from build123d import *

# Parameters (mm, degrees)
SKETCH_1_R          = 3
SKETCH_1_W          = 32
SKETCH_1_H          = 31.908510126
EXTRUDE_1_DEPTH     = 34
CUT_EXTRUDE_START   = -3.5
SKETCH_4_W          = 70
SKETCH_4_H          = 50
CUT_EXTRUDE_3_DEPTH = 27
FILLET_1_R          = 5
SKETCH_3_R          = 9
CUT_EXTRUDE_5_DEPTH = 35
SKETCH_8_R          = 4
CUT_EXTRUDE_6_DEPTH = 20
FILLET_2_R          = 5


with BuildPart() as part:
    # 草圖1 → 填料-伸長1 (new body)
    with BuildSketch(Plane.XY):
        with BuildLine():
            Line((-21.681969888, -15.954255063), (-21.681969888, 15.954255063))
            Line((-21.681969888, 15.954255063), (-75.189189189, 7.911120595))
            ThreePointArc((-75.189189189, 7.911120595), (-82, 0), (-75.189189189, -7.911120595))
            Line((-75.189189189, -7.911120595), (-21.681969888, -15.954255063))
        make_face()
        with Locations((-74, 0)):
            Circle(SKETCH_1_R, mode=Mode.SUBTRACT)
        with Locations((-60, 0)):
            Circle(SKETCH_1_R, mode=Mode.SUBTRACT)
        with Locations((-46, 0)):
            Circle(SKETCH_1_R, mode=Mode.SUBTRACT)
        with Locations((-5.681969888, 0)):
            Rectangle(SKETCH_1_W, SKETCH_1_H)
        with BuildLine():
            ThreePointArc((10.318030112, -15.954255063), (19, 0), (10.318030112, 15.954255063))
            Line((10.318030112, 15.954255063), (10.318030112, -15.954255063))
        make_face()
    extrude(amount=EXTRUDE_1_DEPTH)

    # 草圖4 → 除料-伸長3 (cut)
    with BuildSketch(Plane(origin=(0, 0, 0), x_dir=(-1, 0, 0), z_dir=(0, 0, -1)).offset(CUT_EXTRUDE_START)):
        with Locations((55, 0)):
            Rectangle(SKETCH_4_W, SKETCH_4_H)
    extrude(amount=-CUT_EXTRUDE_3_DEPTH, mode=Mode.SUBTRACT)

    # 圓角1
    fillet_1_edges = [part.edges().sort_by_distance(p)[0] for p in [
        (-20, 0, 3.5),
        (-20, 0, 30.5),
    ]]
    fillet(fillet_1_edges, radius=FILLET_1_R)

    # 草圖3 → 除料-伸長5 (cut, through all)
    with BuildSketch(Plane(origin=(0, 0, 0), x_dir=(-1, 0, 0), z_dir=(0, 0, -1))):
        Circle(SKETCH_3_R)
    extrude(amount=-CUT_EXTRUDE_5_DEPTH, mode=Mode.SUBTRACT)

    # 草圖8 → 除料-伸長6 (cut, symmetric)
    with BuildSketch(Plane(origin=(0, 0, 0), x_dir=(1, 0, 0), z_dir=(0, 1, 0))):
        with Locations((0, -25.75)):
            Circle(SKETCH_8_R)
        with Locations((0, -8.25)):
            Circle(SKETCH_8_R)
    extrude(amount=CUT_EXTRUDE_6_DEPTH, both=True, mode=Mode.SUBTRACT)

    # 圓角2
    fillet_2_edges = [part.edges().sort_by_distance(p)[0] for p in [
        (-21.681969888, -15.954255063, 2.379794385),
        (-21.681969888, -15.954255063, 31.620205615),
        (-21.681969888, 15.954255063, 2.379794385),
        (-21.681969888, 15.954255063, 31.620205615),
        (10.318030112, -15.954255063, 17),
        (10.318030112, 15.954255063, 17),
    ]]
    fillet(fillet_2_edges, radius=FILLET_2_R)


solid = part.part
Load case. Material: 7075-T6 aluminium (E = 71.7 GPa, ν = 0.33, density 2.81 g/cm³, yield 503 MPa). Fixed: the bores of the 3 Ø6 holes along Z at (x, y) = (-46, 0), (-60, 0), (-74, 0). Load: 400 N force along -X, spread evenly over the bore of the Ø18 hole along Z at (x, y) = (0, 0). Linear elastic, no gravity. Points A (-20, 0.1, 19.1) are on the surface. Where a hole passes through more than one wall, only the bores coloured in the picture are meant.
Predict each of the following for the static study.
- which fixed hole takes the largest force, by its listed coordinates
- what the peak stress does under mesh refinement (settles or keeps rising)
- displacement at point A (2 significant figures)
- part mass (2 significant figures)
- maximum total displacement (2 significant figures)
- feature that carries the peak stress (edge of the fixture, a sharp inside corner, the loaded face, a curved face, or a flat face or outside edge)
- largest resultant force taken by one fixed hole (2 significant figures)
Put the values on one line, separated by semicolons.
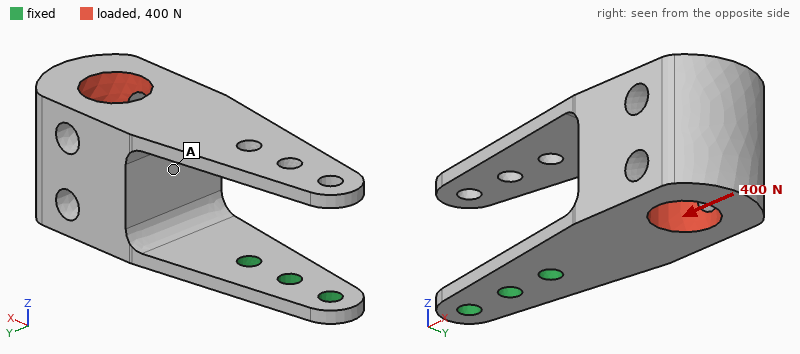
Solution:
(-46, 0); keeps rising; 0.42 mm; 110 g; 1.2 mm; edge of the fixture; 330 N
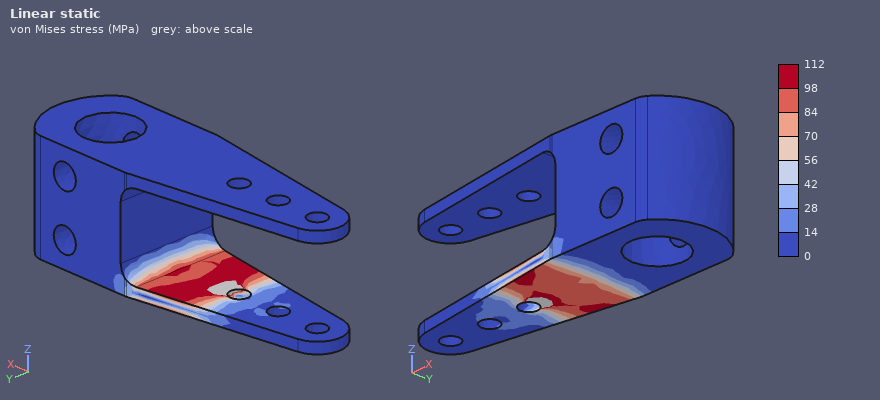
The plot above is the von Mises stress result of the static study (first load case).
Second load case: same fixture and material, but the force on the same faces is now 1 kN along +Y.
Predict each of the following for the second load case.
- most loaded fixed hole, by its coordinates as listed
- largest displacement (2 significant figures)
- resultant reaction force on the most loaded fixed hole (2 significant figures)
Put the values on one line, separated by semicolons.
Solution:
(-46, 0); 1.1 mm; 2.6 kN
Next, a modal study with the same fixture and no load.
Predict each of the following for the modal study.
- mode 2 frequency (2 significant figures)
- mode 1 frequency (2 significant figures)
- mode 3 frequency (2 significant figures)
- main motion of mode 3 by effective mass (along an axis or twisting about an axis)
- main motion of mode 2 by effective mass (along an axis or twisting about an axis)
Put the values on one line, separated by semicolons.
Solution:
540 Hz; 240 Hz; 1000 Hz; along Z; along Y
